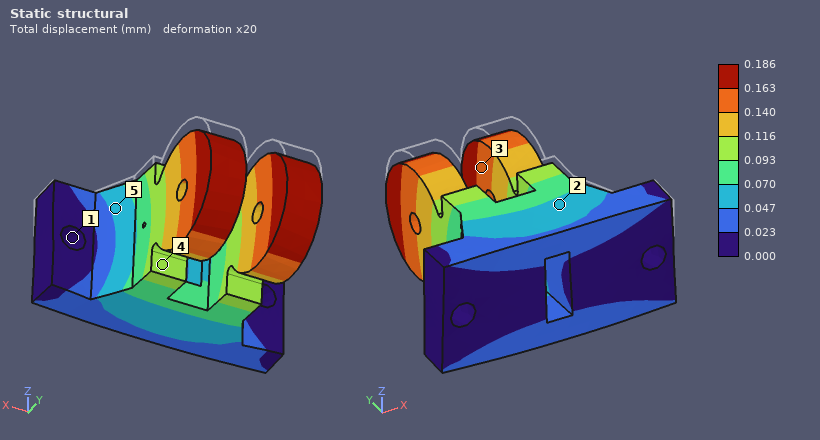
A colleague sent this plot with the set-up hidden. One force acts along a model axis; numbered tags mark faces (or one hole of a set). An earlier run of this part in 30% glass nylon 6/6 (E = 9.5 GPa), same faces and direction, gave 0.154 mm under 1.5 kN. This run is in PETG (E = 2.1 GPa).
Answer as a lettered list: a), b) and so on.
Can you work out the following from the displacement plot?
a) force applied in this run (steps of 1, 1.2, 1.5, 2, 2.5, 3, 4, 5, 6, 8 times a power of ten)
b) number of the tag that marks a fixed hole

a) 400 N
b) 1
